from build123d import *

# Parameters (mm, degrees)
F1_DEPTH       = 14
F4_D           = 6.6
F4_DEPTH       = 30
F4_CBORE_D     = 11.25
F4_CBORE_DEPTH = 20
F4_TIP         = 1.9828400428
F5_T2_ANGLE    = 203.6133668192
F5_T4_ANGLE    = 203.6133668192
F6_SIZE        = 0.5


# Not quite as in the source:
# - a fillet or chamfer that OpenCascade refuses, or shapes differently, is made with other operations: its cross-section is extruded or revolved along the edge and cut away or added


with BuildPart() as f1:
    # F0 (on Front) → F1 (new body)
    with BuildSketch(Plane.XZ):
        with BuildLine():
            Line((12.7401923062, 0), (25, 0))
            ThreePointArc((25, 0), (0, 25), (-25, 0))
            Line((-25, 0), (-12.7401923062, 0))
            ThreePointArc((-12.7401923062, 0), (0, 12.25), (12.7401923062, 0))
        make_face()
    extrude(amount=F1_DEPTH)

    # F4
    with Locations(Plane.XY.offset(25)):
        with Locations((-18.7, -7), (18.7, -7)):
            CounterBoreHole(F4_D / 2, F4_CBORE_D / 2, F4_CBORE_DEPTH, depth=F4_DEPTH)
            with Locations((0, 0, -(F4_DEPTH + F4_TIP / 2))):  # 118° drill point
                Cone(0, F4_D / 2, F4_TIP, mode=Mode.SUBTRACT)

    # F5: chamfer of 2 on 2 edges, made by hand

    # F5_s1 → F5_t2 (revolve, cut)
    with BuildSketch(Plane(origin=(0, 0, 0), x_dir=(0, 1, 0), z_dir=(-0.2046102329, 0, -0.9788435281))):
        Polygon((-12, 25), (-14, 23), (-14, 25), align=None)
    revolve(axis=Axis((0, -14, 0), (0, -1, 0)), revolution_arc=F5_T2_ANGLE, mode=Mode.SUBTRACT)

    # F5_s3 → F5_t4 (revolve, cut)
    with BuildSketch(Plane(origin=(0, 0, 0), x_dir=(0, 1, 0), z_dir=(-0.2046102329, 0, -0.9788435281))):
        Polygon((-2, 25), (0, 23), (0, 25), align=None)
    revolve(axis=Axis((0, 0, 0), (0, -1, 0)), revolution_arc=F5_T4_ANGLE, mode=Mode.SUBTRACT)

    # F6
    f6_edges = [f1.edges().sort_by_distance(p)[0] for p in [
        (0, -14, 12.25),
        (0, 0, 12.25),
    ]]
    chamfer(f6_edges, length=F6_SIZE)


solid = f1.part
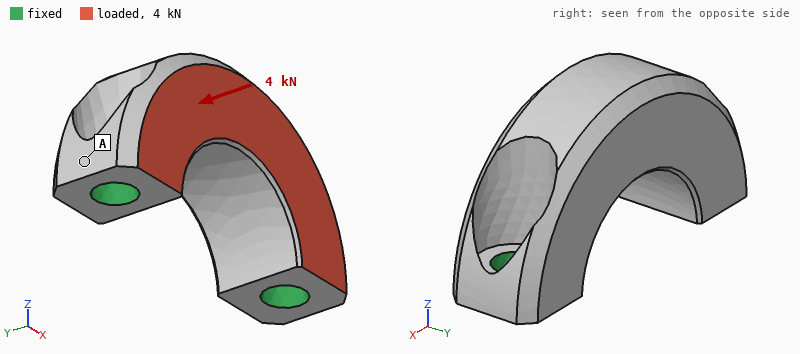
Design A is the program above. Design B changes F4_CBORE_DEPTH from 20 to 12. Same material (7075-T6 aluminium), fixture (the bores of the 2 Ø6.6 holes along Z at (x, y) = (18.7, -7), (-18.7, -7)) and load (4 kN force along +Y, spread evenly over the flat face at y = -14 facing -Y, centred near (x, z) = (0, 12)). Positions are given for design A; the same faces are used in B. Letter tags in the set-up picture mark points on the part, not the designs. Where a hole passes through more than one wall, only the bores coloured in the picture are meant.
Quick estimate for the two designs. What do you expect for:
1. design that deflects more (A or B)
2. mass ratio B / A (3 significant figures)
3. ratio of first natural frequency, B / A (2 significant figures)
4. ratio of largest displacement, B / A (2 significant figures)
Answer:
A
1.13
2.1
0.21
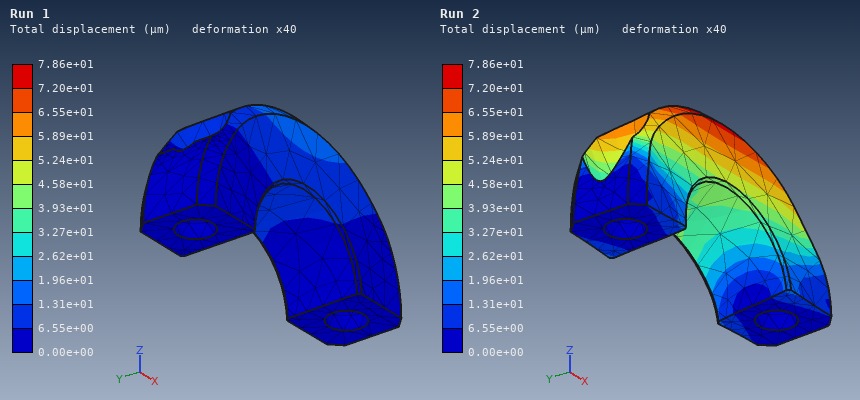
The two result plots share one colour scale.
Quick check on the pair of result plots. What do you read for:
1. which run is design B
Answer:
Run 1
